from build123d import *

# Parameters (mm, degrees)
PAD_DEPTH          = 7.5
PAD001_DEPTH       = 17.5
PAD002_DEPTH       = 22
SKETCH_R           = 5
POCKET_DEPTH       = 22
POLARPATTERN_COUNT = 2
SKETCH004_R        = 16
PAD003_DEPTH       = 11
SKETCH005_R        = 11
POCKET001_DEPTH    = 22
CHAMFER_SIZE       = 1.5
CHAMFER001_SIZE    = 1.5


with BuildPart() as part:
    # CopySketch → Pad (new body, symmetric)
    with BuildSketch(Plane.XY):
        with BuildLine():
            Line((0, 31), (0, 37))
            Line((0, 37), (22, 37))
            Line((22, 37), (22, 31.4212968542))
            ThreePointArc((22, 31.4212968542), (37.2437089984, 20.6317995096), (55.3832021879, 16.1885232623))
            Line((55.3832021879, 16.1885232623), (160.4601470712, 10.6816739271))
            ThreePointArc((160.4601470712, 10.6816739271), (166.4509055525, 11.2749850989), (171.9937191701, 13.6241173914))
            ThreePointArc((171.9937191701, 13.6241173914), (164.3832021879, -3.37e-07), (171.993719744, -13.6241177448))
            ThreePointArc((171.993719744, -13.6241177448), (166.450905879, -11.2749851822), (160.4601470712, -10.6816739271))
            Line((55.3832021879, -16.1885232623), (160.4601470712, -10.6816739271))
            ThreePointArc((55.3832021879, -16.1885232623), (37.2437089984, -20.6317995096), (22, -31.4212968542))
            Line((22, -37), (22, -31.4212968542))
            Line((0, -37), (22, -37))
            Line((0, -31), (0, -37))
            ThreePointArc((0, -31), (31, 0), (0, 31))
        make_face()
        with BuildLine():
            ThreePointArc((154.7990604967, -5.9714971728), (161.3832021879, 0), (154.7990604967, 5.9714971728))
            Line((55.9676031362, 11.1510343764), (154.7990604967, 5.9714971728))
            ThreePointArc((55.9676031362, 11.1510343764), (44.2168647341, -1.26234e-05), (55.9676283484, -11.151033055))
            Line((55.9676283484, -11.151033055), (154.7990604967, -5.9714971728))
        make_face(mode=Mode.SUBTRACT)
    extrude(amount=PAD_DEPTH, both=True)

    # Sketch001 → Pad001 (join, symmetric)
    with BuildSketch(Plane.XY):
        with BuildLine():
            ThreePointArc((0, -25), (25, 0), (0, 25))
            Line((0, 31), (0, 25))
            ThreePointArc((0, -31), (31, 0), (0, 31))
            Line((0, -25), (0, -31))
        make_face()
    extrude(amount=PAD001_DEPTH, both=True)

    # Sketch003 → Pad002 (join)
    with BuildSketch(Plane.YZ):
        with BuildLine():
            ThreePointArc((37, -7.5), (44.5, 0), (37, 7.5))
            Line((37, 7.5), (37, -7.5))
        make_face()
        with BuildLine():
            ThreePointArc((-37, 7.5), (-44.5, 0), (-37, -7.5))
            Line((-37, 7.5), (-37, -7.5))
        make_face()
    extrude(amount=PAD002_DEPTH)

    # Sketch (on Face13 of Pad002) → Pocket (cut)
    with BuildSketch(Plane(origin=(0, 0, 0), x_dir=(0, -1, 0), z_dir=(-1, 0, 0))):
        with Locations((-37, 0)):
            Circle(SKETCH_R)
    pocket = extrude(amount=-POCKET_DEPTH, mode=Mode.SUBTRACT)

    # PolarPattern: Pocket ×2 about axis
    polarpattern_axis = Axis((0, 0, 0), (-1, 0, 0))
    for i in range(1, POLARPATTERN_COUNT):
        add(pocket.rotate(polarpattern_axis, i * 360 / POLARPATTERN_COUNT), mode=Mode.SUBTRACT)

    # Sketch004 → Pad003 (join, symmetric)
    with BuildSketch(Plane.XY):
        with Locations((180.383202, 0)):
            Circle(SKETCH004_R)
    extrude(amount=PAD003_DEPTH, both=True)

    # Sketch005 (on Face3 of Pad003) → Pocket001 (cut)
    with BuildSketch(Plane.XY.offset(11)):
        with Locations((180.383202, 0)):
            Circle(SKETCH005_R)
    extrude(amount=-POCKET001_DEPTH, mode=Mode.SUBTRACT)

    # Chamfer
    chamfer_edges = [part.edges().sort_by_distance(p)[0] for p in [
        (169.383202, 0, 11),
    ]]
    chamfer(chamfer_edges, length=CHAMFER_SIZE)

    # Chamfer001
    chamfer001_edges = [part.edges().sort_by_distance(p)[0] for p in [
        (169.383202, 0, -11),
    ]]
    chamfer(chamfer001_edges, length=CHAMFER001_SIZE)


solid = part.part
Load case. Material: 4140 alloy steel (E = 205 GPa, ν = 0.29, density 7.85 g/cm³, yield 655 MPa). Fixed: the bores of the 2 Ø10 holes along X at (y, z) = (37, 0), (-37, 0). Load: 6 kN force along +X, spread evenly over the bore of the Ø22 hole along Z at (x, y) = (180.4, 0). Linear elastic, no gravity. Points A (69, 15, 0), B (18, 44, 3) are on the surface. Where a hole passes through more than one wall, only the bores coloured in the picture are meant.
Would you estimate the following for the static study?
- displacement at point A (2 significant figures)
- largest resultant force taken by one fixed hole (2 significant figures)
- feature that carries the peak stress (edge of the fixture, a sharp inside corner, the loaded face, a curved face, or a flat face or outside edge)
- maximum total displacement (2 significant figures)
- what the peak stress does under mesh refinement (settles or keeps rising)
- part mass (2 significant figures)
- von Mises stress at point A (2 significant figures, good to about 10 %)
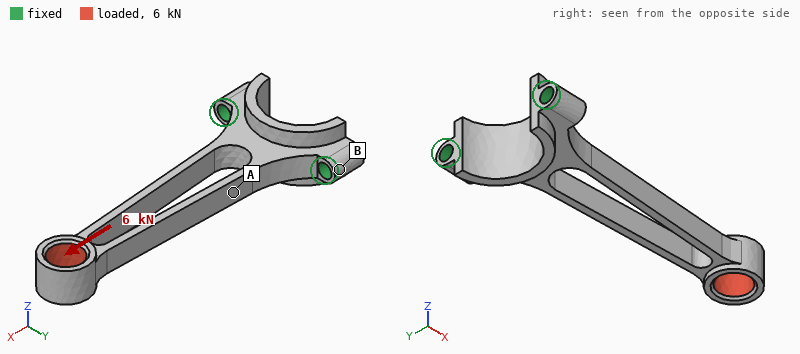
9.3 µm
3.6 kN
a sharp inside corner
37 µm
keeps rising
520 g
36 MPa
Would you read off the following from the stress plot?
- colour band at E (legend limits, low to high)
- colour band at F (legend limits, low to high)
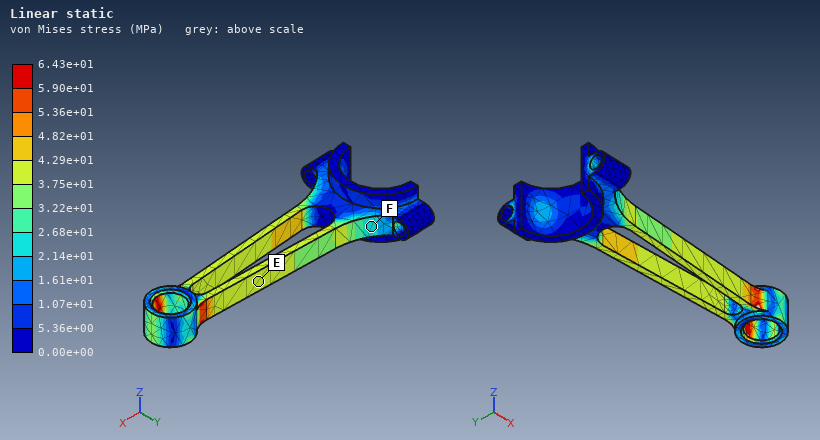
3.75e+01 to 4.29e+01 MPa
2.14e+01 to 2.68e+01 MPa
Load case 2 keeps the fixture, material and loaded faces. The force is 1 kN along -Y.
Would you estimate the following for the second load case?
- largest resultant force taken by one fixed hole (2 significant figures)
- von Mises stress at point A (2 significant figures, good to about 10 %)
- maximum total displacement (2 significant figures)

3.3 kN
220 MPa
1.0 mm
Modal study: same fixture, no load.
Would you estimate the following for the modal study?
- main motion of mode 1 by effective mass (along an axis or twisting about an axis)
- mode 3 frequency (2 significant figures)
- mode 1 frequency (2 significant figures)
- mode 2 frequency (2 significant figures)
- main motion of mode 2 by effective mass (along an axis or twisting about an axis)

along Z
1400 Hz
370 Hz
420 Hz
along Y
